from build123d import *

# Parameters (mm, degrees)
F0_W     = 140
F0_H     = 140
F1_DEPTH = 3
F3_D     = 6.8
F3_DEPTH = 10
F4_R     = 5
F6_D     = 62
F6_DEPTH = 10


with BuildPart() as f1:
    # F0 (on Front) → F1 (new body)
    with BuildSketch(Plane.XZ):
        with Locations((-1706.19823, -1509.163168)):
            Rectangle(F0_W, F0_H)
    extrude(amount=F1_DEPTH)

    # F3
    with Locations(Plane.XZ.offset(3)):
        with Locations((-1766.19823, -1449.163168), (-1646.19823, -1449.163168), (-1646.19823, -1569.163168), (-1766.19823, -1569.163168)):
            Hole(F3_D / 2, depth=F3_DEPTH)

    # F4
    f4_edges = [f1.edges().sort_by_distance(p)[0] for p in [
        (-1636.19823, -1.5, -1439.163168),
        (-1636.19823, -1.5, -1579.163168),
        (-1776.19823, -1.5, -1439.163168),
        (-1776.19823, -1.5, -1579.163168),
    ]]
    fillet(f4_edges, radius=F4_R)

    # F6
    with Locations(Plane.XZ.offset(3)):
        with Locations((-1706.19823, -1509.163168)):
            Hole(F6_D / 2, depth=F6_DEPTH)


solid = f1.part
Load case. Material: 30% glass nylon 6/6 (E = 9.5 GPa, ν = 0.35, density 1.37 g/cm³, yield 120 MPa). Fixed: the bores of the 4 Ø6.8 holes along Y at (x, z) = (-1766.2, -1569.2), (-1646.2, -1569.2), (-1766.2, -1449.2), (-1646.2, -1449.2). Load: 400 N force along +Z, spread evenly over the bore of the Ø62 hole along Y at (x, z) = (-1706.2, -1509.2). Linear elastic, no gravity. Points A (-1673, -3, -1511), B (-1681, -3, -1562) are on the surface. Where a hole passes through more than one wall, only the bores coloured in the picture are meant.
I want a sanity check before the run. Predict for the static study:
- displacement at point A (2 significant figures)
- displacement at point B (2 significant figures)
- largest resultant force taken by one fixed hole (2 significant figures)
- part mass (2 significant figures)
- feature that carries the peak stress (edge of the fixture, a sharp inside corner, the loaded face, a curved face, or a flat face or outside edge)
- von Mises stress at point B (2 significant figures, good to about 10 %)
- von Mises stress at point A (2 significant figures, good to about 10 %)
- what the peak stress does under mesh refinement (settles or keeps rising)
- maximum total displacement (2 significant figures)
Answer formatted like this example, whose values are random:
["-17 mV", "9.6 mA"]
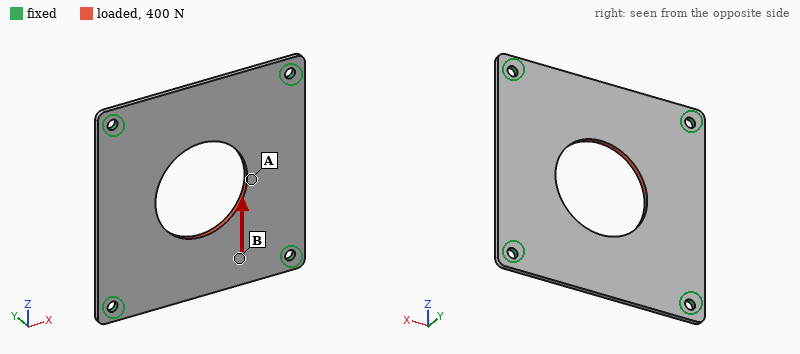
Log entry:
["7.2 µm", "8.1 µm", "110 N", "67 g", "edge of the fixture", "0.67 MPa", "1.3 MPa", "keeps rising", "12 µm"]
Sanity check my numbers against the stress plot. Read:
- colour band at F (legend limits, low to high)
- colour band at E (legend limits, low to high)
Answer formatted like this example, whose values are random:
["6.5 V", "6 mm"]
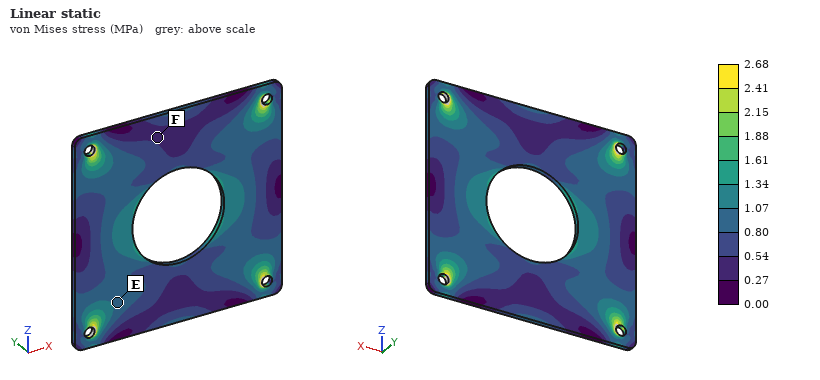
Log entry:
["0.27 to 0.54 MPa", "0.80 to 1.07 MPa"]
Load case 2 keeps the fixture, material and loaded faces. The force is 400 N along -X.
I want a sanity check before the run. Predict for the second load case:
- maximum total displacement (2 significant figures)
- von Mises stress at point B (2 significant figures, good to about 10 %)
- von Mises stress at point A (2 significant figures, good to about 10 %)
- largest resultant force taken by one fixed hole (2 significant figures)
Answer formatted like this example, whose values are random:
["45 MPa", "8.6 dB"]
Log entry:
["12 µm", "0.77 MPa", "0.74 MPa", "110 N"]
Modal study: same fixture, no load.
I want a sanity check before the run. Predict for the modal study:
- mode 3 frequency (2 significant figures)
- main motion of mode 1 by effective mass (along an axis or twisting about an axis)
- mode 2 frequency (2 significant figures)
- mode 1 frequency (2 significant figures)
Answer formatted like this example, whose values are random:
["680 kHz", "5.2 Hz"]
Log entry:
["620 Hz", "along Y", "620 Hz", "430 Hz"]
